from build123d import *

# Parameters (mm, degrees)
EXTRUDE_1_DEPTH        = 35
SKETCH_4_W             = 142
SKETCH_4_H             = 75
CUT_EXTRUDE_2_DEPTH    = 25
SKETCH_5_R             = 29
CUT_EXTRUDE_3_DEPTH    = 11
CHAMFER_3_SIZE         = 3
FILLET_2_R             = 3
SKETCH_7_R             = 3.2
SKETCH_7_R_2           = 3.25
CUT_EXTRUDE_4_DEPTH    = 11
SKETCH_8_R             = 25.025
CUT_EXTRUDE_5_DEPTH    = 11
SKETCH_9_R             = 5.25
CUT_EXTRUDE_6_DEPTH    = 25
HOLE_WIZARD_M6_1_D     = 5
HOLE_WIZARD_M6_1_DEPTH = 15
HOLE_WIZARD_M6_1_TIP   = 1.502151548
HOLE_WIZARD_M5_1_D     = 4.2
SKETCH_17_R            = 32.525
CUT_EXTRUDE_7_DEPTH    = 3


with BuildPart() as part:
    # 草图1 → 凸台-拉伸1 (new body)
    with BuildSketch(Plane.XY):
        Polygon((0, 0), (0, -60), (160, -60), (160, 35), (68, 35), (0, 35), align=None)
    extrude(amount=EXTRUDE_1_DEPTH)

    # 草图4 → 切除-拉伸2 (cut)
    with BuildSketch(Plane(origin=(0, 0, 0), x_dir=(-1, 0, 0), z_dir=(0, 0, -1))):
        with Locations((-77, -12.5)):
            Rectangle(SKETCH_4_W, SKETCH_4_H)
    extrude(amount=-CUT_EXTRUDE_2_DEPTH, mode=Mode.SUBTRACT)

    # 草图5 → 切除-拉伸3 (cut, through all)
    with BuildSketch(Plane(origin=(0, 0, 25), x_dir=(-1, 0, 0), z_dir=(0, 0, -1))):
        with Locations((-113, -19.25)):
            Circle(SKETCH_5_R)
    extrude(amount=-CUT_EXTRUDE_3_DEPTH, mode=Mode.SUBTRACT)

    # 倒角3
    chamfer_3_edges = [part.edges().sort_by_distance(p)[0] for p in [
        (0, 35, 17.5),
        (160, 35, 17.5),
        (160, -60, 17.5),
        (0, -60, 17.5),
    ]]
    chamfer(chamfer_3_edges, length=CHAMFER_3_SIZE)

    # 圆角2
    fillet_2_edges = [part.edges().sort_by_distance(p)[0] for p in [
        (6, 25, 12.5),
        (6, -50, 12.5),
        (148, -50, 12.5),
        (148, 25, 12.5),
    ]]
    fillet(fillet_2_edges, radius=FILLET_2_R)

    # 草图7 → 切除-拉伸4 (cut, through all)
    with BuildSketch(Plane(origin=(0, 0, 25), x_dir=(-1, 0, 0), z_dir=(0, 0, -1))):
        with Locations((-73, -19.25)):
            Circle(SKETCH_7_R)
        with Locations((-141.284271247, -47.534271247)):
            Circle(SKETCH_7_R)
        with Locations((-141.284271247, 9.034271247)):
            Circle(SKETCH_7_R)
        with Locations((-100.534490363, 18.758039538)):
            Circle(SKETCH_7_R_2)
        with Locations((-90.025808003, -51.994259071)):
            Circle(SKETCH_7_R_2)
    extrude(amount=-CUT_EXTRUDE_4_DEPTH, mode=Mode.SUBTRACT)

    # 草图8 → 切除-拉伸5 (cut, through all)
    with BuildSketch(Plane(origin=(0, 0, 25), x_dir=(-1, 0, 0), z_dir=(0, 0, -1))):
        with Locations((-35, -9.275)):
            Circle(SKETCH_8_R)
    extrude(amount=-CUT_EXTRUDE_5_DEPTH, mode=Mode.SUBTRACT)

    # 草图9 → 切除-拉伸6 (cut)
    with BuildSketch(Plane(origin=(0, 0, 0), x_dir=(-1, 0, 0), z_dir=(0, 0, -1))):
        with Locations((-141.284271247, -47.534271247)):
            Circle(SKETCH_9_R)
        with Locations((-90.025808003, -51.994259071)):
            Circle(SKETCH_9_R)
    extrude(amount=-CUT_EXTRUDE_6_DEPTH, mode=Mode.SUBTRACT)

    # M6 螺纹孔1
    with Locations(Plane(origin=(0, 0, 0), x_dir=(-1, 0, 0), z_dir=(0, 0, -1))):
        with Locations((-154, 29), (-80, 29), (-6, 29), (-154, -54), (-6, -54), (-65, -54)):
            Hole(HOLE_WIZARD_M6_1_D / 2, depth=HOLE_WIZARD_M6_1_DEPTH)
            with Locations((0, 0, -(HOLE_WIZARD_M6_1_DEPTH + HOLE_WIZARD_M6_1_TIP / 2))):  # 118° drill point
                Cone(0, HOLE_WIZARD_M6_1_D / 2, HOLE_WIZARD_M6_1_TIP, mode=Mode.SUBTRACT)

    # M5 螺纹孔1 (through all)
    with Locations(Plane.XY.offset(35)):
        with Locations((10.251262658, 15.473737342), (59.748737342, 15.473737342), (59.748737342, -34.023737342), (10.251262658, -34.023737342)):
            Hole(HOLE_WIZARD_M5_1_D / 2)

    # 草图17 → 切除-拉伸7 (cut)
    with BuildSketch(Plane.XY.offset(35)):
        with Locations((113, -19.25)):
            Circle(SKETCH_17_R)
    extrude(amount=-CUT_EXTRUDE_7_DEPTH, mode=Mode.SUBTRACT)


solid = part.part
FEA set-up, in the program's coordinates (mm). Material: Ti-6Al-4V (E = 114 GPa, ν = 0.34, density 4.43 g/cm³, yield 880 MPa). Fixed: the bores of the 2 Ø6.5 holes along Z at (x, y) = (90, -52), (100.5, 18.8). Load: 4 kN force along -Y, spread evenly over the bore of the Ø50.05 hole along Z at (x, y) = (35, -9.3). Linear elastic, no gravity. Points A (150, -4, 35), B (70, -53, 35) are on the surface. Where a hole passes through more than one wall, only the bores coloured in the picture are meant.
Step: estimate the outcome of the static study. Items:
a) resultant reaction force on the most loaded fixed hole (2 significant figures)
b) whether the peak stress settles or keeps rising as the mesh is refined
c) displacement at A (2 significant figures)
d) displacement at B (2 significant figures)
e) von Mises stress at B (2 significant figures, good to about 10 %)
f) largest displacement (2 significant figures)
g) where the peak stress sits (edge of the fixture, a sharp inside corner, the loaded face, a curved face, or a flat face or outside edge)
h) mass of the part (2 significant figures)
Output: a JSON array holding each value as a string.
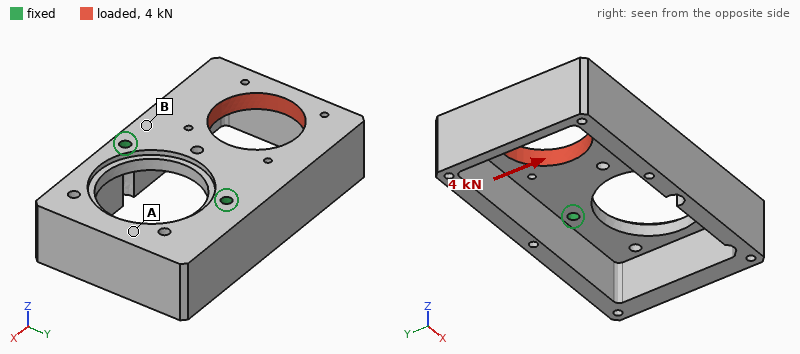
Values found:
["3.8 kN", "keeps rising", "6.1 µm", "6.7 µm", "11 MPa", "40 µm", "edge of the fixture", "940 g"]
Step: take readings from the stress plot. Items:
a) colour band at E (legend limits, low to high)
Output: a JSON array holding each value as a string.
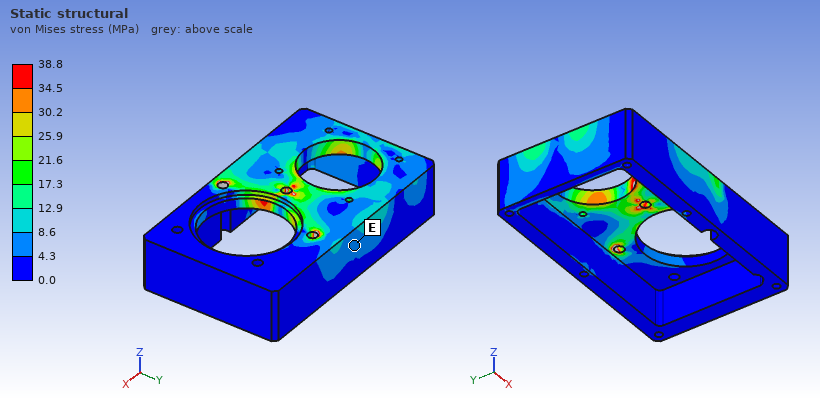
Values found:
["4.3 to 8.6 MPa"]
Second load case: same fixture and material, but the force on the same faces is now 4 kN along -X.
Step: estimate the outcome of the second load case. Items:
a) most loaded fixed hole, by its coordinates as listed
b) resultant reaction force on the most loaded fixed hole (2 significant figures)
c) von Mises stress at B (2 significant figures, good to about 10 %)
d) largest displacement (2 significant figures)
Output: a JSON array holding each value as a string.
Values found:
["(100.5, 18.8)", "2.4 kN", "7.0 MPa", "12 µm"]
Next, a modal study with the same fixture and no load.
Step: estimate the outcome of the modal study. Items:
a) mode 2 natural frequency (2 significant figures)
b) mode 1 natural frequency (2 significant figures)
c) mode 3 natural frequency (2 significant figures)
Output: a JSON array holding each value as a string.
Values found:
["1600 Hz", "890 Hz", "2400 Hz"]
